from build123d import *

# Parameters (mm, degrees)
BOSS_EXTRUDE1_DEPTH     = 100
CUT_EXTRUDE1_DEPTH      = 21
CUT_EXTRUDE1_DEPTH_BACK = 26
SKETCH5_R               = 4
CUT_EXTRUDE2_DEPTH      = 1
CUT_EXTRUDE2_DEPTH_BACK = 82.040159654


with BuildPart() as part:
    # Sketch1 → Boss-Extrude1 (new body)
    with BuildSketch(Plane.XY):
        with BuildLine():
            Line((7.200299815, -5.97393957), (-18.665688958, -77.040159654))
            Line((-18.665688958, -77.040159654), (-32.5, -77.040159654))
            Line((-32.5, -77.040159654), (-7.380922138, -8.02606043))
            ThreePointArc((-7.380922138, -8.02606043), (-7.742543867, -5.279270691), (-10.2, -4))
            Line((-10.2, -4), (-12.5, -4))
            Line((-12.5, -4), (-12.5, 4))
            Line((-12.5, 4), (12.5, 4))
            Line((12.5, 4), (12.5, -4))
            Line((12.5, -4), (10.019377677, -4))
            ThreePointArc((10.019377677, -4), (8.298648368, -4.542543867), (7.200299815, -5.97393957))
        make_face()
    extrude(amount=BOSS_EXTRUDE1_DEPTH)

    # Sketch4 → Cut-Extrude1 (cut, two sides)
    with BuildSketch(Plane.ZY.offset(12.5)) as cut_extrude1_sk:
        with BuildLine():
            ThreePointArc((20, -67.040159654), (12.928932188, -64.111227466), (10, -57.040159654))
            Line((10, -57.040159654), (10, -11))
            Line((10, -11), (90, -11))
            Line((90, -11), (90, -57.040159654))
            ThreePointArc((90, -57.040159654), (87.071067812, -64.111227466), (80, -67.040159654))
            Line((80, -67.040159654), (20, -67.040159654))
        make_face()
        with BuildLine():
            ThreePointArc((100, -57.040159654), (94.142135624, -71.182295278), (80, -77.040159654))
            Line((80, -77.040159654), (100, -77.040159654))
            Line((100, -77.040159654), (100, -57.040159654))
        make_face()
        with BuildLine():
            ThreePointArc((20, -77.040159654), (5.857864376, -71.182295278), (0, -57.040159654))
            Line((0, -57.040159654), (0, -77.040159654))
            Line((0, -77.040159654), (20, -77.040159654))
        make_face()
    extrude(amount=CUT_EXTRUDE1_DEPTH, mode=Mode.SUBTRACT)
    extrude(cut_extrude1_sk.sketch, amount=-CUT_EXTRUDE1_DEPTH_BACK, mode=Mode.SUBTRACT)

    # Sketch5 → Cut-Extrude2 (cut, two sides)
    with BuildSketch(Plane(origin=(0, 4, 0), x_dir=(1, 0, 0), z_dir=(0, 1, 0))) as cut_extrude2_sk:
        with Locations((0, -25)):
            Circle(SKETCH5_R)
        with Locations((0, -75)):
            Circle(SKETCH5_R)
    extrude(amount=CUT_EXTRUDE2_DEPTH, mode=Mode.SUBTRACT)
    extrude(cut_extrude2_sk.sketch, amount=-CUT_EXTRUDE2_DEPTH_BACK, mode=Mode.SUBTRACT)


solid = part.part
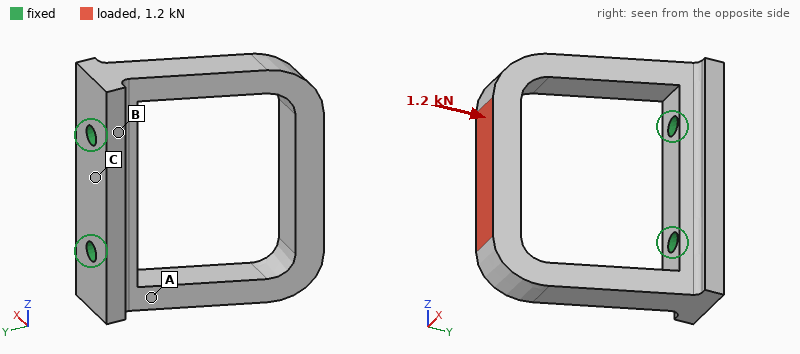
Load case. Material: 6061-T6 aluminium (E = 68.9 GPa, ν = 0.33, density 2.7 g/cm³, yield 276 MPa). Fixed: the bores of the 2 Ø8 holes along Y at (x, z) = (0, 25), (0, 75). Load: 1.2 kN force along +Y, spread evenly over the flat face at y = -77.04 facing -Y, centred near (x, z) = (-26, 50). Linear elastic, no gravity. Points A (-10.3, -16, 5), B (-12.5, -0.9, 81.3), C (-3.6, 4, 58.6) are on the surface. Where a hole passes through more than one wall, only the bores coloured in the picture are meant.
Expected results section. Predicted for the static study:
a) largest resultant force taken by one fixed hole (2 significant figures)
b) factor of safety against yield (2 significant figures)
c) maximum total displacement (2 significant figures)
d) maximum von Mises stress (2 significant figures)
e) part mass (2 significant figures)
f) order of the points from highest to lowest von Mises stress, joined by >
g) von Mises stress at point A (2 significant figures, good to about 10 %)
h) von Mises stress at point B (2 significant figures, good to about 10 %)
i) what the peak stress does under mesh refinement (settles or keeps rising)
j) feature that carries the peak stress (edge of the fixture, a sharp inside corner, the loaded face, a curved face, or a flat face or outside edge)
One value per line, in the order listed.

650 N
3.4
0.40 mm
81 MPa
150 g
A > B > C
50 MPa
14 MPa
settles
a curved face
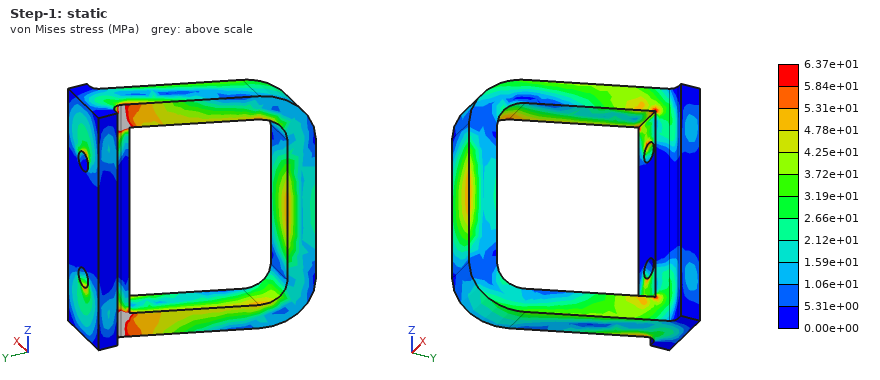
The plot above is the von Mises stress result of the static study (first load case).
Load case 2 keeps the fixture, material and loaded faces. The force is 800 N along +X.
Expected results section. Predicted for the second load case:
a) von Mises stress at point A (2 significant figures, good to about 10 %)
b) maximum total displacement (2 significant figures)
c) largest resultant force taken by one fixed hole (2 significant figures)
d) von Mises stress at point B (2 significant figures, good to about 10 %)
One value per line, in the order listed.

81 MPa
0.66 mm
400 N
26 MPa
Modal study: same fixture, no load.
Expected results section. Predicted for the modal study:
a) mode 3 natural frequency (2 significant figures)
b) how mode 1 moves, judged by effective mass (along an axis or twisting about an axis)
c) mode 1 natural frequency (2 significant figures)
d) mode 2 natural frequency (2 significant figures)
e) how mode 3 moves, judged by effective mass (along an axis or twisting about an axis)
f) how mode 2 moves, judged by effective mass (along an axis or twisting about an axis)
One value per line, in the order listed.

2000 Hz
along X
970 Hz
1400 Hz
twisting about Y
along Z
